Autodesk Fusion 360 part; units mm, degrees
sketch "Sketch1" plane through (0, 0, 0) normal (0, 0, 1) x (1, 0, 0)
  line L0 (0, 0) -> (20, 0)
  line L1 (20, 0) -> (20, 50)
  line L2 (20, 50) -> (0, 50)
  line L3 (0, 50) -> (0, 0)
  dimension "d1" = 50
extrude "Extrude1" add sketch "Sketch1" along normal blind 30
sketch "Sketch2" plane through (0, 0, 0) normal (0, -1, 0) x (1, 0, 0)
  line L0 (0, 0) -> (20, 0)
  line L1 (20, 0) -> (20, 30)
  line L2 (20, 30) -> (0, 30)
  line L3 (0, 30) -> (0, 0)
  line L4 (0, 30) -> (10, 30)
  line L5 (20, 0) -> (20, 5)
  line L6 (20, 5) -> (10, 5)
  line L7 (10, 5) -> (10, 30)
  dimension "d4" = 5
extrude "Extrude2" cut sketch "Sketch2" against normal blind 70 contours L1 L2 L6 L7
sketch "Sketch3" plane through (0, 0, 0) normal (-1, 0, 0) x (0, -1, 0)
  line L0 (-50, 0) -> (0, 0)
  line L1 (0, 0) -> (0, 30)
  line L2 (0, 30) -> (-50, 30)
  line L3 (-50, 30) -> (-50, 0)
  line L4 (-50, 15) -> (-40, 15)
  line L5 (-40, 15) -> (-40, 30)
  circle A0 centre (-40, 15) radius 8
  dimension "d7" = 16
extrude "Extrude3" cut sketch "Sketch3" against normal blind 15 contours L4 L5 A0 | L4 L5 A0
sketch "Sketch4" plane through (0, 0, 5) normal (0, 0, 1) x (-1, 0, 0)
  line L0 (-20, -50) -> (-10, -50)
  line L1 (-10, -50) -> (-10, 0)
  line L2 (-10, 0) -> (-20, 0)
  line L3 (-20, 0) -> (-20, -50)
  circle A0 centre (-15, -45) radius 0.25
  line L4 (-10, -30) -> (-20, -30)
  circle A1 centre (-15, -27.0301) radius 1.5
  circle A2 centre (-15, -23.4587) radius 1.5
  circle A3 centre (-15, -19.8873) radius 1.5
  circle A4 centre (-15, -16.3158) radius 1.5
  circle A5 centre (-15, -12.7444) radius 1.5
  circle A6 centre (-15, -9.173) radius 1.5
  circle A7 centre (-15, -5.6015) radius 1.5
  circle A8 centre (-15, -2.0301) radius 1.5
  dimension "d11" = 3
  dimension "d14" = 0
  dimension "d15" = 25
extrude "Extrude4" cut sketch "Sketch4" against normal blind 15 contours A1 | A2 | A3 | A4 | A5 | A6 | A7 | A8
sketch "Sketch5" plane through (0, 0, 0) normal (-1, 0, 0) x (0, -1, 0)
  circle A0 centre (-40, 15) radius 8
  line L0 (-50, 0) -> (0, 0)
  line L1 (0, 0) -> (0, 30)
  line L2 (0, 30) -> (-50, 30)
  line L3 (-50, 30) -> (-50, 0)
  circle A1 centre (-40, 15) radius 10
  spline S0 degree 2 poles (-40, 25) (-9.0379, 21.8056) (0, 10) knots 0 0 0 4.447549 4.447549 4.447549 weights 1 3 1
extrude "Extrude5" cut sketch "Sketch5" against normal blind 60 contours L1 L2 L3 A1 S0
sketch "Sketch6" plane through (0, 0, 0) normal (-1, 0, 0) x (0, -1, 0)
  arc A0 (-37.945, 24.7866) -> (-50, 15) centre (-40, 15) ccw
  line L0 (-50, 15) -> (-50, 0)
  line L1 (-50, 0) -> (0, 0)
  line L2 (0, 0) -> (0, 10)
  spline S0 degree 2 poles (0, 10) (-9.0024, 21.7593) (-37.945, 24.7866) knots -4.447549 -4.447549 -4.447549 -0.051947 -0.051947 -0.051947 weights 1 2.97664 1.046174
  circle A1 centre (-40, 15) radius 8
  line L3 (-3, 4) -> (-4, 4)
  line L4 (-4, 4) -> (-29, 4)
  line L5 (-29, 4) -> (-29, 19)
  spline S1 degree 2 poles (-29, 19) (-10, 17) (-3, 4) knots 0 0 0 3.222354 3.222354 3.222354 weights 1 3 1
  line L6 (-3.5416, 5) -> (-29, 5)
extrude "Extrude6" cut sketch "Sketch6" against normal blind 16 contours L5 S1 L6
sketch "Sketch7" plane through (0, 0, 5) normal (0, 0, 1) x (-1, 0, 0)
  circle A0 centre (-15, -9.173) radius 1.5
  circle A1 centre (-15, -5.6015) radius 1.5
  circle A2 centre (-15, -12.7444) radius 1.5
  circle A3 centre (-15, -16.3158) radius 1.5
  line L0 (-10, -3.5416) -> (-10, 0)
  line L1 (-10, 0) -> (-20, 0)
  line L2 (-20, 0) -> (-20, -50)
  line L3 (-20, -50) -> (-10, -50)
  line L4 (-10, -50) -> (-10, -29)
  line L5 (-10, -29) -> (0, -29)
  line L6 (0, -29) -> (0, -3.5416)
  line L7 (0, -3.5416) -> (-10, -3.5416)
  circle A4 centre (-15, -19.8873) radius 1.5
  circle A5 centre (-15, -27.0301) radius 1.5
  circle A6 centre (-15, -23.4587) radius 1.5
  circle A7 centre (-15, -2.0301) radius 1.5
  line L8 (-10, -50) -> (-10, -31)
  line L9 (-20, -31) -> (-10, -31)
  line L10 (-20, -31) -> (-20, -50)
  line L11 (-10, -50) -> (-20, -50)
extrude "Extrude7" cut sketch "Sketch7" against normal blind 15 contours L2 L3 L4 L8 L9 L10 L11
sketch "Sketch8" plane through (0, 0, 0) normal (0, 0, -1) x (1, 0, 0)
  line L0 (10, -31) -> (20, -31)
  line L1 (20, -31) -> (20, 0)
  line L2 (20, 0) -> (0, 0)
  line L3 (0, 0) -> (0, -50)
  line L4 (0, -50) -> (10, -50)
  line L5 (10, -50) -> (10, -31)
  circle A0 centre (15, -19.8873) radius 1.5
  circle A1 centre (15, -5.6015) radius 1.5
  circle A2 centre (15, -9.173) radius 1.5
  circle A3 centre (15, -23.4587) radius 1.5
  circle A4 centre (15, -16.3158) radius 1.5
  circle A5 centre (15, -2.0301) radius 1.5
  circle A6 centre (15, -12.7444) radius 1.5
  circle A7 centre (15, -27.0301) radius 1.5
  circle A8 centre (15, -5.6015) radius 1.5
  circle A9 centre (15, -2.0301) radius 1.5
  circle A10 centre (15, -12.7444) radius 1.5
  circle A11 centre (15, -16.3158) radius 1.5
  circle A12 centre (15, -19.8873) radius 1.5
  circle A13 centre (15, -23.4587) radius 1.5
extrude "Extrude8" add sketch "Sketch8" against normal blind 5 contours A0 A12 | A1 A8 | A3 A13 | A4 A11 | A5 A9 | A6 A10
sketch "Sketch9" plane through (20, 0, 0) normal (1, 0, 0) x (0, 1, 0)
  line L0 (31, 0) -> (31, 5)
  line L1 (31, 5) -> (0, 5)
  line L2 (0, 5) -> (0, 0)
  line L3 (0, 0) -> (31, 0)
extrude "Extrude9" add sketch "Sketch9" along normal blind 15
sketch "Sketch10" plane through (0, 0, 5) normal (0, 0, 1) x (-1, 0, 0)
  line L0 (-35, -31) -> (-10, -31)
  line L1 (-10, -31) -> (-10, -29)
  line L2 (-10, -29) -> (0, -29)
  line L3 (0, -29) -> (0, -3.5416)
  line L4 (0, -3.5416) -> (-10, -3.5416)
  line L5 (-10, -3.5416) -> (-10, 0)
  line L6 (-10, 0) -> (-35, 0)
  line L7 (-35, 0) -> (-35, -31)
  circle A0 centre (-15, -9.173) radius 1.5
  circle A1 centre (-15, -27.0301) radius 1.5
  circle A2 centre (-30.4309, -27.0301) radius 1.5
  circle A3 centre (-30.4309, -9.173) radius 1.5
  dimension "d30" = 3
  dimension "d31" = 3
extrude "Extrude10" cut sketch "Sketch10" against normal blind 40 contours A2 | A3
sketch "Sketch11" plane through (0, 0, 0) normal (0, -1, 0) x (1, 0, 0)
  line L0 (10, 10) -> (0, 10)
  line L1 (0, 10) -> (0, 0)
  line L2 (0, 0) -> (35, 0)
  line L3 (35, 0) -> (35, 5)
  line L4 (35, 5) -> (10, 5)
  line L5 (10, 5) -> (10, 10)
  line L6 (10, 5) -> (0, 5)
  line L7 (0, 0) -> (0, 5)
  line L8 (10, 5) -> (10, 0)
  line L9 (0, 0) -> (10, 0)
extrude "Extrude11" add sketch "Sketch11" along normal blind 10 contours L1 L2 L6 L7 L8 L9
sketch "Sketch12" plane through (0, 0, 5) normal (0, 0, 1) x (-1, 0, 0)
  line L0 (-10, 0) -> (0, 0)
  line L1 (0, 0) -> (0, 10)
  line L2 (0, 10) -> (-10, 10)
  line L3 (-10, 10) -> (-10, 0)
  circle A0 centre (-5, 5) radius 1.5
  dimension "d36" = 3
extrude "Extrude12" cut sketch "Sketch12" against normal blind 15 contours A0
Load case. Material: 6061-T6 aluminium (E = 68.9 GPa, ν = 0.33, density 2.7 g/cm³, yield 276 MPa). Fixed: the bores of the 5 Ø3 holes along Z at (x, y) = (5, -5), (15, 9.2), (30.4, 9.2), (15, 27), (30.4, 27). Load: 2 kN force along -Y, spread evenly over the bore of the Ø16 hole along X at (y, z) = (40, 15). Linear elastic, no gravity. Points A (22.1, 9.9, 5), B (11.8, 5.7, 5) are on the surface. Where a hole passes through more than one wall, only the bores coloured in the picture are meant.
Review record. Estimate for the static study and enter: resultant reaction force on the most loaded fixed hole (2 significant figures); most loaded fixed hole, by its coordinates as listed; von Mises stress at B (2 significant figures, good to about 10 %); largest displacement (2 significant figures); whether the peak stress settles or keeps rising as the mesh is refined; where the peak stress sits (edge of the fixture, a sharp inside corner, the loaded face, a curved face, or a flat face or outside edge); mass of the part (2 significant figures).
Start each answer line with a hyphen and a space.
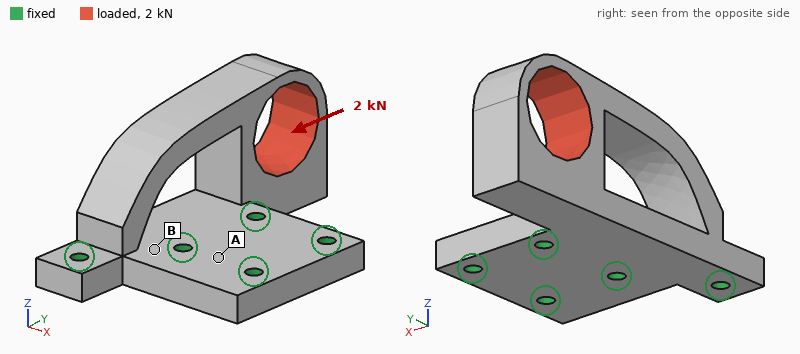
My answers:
- 1.2 kN
- (5, -5)
- 27 MPa
- 0.15 mm
- keeps rising
- edge of the fixture
- 28 g
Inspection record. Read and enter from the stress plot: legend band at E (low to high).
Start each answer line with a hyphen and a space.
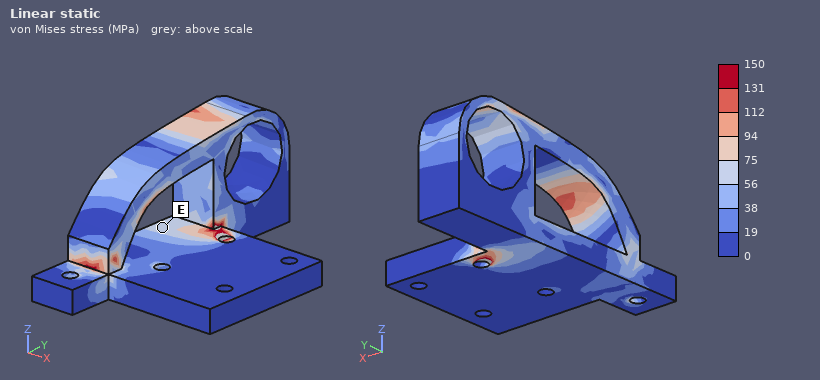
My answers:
- 56 to 75 MPa
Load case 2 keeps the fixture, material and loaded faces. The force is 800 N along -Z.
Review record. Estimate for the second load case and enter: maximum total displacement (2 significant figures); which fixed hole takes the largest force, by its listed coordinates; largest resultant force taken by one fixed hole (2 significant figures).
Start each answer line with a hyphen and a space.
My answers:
- 0.15 mm
- (15, 27)
- 1.2 kN
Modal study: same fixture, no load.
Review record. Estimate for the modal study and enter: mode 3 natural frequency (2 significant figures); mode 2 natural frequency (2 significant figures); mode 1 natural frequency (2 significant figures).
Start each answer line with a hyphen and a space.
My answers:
- 9400 Hz
- 6500 Hz
- 4100 Hz
